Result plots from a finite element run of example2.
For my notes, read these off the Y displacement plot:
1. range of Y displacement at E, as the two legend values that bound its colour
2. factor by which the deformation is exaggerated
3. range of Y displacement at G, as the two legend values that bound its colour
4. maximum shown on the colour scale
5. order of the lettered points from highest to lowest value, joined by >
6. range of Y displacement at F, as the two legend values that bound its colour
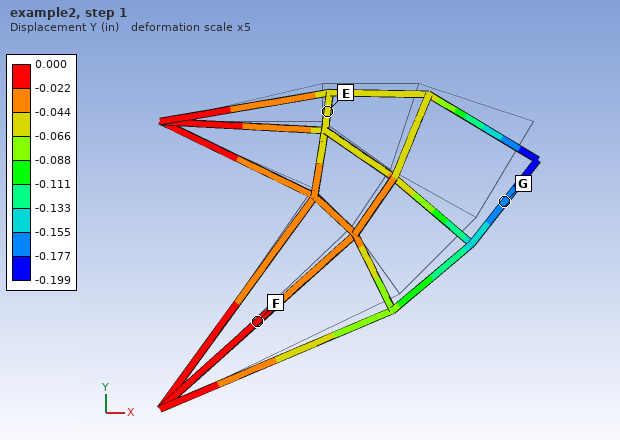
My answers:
-0.066 to -0.044 in
5
-0.177 to -0.155 in
0.000 in
F > E > G
-0.022 to 0.000 in
